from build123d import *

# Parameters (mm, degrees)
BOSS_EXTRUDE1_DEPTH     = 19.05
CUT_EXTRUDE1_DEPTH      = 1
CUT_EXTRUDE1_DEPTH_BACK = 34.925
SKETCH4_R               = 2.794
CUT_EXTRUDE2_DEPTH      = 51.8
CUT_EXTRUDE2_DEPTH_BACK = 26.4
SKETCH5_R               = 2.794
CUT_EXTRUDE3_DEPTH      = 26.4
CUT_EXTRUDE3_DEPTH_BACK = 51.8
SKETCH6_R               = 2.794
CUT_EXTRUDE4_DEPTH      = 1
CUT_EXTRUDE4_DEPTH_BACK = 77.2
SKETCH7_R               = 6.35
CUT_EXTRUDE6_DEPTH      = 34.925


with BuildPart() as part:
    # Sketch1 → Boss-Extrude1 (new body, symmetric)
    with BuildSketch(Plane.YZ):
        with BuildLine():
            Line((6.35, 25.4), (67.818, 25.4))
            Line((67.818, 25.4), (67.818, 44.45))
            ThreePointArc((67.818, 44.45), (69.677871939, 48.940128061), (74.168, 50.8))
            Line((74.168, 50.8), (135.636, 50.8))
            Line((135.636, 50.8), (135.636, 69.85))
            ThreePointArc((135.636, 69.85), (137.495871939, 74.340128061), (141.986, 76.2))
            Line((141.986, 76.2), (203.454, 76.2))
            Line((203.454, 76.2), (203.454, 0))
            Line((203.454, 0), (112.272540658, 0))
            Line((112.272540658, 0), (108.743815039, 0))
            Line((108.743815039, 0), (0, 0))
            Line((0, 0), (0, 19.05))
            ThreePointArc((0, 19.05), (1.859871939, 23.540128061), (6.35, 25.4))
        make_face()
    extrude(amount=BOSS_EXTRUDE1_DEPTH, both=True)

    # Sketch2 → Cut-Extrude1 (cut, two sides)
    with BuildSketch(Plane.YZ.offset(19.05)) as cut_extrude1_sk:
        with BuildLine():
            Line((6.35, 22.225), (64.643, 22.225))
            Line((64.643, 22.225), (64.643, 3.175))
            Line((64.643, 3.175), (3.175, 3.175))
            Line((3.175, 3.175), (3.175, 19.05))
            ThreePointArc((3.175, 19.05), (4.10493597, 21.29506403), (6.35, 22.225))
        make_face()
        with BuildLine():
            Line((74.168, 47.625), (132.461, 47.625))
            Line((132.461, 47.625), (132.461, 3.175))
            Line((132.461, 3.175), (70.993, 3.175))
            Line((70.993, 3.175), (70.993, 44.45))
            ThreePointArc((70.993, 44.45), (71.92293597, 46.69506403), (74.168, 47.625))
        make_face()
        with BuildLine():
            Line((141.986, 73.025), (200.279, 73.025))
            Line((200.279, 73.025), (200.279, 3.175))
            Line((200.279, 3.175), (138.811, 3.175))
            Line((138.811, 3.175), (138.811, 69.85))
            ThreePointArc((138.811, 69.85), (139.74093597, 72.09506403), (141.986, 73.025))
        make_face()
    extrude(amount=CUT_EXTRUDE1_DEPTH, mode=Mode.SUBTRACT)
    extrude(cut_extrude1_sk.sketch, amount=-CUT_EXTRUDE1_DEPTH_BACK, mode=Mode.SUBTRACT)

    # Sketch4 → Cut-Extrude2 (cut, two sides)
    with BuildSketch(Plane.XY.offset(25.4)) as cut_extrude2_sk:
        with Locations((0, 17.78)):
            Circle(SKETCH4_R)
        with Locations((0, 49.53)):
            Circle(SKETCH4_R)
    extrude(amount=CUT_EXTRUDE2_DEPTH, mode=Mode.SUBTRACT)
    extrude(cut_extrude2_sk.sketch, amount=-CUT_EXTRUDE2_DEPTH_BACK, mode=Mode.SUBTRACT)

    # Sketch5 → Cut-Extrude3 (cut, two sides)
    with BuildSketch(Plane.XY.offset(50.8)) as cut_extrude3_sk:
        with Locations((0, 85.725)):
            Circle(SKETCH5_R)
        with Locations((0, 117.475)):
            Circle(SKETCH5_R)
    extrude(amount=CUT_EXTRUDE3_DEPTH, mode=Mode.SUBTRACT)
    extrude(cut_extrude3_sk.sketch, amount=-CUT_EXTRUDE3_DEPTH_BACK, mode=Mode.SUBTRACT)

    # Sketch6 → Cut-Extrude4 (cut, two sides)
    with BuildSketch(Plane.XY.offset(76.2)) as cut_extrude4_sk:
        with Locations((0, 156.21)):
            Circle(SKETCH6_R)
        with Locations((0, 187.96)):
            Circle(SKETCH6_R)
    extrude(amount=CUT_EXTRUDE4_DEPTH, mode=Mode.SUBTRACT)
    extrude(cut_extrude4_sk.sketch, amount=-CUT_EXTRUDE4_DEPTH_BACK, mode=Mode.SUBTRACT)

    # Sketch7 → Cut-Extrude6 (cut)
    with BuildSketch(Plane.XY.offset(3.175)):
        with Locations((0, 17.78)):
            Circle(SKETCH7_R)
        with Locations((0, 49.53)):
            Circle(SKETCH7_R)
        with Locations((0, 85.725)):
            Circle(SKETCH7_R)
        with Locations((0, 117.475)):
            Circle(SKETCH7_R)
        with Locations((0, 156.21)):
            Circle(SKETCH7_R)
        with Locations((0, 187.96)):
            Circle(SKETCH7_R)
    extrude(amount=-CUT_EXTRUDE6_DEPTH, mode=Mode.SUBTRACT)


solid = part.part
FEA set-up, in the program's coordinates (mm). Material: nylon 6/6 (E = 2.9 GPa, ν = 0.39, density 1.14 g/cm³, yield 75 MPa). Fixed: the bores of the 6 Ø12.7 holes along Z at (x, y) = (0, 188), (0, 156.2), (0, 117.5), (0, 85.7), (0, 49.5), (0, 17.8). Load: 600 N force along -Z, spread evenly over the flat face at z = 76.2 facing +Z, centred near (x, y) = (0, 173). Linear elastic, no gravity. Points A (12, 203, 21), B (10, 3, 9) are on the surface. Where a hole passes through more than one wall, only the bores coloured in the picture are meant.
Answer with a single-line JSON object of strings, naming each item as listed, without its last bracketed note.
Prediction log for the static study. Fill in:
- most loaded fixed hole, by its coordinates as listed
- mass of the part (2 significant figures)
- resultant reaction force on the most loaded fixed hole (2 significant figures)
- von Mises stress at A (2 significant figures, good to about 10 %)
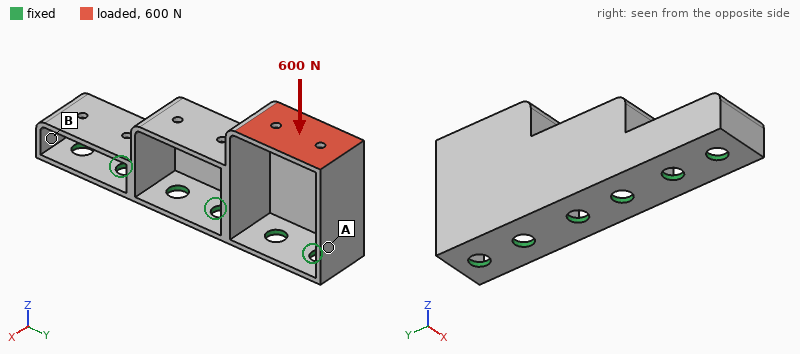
{"most loaded fixed hole, by its coordinates as listed": "(0, 188)", "mass of the part": "120 g", "resultant reaction force on the most loaded fixed hole": "310 N", "von Mises stress at A": "4.7 MPa"}
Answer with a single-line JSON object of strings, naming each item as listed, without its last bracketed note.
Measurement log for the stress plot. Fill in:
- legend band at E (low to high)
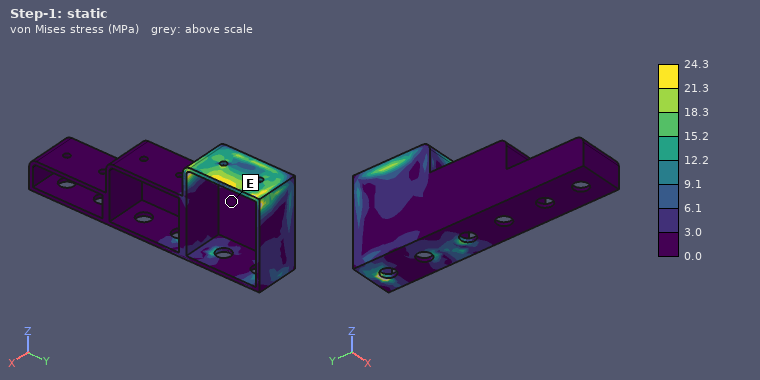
{"legend band at E": "0.0 to 3.0 MPa"}
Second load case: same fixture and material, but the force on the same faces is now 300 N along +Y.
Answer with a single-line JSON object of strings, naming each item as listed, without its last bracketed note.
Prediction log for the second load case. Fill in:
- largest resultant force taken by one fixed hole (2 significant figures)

{"largest resultant force taken by one fixed hole": "140 N"}
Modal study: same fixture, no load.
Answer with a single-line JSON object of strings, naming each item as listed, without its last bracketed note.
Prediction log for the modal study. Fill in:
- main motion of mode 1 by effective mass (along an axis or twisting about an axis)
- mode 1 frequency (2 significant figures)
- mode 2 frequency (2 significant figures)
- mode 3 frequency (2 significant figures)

{"main motion of mode 1 by effective mass": "along X", "mode 1 frequency": "290 Hz", "mode 2 frequency": "500 Hz", "mode 3 frequency": "850 Hz"}
